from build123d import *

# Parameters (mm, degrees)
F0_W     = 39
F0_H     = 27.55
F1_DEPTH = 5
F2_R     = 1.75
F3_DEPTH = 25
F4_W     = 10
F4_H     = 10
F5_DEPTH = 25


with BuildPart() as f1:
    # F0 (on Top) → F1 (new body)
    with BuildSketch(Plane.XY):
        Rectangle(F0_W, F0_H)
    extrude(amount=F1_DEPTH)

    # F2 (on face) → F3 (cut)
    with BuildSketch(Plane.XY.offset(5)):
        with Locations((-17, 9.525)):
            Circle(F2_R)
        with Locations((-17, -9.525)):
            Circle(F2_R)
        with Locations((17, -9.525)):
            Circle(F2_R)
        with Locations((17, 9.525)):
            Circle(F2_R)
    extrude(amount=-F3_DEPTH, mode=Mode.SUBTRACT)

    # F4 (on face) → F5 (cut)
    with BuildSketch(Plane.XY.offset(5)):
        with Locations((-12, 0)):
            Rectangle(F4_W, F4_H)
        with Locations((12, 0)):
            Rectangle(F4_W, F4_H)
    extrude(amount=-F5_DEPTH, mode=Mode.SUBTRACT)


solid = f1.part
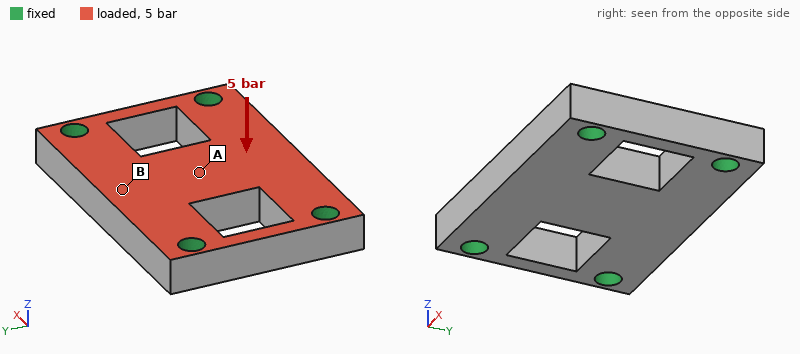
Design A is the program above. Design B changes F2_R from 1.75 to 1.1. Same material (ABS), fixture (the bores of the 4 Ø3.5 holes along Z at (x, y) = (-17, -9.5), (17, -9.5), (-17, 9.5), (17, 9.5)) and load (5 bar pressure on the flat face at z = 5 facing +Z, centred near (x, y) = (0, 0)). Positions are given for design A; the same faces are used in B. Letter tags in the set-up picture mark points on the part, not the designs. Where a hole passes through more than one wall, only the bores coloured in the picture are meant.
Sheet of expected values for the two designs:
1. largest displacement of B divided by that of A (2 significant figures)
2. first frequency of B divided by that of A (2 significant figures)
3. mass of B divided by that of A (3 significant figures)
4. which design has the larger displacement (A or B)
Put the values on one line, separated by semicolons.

1.2; 0.90; 1.03; B
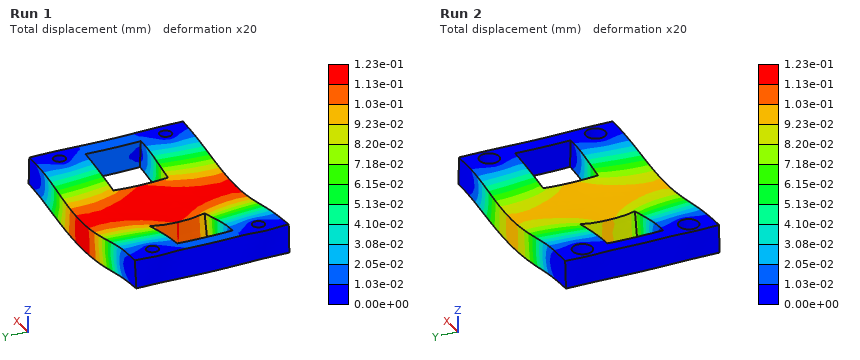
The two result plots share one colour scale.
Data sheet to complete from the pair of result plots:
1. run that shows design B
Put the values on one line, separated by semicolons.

Run 1
